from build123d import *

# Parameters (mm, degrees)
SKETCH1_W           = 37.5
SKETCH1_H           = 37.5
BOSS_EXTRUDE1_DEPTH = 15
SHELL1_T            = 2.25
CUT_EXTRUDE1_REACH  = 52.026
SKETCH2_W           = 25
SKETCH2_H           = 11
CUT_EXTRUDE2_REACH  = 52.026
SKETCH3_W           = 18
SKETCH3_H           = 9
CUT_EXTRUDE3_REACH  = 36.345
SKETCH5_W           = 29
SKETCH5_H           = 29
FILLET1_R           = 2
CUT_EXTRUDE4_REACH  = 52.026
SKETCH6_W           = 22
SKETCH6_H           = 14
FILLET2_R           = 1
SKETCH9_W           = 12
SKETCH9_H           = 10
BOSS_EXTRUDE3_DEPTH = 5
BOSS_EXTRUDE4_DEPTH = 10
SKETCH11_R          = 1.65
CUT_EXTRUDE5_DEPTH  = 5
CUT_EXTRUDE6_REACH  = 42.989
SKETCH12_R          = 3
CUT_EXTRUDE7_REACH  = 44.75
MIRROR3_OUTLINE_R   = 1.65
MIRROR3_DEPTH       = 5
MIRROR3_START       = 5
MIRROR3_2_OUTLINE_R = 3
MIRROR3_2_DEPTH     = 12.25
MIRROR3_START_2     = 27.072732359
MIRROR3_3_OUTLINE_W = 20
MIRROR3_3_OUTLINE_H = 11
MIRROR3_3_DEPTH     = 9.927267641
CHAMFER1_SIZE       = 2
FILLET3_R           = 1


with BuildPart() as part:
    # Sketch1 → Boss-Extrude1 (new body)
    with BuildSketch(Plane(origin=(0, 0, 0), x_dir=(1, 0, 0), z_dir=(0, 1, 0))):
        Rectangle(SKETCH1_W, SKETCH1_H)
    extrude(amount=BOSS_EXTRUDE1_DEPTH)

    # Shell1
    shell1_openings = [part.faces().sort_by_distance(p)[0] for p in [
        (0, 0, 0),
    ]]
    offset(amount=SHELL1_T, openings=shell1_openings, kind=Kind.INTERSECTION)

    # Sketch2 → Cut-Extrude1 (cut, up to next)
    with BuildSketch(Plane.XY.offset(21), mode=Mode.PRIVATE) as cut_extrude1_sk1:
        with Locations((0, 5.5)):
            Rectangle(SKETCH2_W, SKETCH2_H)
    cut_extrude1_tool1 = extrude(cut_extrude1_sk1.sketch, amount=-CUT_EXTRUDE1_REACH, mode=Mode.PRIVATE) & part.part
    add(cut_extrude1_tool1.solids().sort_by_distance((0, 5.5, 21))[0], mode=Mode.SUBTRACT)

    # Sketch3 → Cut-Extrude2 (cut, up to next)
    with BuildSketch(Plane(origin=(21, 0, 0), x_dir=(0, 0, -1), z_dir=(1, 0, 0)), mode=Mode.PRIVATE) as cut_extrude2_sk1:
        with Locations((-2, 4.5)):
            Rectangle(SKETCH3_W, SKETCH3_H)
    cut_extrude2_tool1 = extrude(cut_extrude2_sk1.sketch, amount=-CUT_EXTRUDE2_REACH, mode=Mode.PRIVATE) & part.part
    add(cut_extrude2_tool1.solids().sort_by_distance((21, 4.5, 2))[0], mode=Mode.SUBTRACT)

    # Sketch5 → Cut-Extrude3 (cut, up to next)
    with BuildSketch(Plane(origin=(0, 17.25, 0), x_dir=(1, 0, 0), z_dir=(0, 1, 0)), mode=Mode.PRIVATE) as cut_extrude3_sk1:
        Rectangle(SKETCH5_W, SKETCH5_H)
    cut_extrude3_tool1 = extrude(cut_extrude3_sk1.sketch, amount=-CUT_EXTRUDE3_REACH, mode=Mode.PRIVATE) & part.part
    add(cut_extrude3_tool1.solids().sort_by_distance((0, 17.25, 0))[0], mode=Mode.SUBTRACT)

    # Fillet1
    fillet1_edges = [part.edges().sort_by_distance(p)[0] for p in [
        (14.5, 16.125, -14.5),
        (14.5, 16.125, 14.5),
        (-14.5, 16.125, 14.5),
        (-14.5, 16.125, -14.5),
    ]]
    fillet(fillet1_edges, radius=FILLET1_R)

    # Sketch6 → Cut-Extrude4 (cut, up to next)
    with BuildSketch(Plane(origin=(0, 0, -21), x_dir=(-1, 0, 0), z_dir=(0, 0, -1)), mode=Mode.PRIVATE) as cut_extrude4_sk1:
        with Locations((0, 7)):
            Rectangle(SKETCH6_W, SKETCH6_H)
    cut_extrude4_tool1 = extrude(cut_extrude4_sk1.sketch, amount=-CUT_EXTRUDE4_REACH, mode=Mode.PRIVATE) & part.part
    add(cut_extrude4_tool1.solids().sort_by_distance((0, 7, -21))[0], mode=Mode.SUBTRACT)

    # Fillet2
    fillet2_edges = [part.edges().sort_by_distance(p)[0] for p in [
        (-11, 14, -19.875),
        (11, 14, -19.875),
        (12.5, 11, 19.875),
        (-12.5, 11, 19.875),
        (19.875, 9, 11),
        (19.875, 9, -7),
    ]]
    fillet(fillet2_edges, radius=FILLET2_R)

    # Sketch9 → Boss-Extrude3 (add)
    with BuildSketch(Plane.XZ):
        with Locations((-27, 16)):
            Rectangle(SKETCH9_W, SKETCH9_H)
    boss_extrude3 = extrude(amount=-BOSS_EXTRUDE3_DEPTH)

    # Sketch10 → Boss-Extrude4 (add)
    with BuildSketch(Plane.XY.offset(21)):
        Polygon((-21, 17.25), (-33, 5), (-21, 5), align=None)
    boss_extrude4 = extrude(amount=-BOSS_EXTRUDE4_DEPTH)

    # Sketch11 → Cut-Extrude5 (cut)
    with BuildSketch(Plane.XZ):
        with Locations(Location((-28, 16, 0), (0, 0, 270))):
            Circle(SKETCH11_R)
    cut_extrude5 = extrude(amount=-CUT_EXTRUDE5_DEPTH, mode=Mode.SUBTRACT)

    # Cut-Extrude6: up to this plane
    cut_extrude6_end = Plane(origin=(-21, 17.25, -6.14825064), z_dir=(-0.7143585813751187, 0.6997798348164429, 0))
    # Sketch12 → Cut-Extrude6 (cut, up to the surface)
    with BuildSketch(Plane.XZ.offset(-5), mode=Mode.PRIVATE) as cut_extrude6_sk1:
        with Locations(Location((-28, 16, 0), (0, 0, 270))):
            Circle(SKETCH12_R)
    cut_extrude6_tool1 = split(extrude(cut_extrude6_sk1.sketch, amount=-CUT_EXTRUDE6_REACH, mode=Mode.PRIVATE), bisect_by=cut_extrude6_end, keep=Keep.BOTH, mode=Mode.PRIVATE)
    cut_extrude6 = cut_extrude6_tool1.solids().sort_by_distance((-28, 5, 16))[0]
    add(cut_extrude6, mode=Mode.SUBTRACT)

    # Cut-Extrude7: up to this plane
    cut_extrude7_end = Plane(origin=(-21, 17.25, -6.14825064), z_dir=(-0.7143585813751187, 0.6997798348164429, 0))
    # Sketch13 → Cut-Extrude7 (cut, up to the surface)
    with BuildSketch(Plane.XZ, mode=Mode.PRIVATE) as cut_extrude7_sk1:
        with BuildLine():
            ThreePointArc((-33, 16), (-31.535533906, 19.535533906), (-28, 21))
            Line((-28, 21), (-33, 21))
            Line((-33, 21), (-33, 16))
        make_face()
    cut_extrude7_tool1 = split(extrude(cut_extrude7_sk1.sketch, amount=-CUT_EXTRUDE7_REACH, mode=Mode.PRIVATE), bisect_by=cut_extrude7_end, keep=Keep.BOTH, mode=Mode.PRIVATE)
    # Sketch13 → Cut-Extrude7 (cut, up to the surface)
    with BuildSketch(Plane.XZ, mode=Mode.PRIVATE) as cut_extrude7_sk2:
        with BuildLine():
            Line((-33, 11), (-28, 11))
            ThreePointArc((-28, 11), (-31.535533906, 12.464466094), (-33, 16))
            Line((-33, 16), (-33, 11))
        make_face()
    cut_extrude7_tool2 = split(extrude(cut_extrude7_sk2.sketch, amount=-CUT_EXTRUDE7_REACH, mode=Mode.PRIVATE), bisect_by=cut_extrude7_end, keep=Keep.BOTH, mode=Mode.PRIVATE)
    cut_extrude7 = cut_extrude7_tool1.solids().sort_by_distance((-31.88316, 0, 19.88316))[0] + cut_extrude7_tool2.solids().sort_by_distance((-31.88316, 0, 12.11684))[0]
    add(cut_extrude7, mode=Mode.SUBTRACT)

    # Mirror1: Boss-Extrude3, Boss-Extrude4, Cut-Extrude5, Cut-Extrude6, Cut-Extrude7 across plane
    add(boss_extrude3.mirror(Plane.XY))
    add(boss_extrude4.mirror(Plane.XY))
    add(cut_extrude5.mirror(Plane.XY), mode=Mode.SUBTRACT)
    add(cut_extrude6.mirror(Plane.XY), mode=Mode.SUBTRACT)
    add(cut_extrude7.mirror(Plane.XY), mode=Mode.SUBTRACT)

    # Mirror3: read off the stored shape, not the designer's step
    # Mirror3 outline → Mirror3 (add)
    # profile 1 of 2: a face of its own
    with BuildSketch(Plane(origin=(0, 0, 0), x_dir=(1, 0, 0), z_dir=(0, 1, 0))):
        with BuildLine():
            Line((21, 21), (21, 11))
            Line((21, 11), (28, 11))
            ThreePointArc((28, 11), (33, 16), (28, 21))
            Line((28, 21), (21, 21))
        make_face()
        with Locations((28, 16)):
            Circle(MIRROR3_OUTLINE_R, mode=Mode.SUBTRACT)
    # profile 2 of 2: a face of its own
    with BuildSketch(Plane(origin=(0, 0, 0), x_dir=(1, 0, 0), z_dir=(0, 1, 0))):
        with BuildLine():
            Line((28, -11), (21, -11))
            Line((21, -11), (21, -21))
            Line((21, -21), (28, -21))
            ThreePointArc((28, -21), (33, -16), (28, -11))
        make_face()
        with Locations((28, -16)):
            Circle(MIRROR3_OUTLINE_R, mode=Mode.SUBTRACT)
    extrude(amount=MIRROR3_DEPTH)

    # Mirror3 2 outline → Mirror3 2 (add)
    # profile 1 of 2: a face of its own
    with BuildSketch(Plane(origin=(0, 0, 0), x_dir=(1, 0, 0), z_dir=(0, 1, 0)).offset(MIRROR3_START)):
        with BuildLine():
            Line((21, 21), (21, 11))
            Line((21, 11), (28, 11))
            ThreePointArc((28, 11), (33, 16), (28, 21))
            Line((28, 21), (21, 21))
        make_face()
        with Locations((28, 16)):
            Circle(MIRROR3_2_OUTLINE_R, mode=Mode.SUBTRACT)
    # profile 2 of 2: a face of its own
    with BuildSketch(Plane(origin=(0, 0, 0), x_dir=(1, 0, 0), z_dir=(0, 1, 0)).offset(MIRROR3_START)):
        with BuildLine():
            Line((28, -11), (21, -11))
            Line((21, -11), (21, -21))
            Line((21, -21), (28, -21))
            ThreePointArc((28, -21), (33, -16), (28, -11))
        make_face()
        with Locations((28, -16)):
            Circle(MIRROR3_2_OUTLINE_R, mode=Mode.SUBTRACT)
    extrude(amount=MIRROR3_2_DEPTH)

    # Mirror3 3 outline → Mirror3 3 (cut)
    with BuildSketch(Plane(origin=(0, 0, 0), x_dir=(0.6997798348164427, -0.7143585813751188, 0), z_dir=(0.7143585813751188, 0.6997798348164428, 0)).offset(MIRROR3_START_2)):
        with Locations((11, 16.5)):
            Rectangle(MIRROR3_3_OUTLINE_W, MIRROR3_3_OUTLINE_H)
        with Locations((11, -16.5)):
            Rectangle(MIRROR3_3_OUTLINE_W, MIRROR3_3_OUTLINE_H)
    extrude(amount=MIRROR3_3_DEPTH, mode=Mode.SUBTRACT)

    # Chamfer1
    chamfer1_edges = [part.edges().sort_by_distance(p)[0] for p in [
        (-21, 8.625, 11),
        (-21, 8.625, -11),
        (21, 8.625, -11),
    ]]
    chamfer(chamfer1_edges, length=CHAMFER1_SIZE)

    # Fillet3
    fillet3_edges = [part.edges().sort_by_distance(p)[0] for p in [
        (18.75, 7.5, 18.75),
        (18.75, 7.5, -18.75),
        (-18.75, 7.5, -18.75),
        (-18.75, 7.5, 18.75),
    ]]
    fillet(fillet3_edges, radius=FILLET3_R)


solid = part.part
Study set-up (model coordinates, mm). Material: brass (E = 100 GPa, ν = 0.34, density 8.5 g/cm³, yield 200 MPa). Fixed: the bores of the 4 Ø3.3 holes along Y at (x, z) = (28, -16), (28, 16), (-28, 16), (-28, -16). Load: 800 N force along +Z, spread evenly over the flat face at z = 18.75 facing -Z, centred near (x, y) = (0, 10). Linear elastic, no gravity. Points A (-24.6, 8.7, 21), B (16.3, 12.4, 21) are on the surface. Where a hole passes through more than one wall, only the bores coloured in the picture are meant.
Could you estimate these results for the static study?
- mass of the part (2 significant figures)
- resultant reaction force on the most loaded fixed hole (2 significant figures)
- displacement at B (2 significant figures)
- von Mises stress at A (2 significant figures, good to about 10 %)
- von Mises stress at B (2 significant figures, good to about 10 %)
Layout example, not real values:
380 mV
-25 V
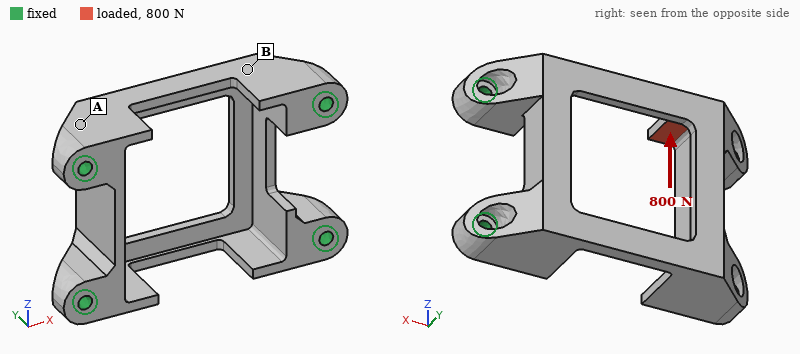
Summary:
87 g
250 N
10 µm
10 MPa
31 MPa
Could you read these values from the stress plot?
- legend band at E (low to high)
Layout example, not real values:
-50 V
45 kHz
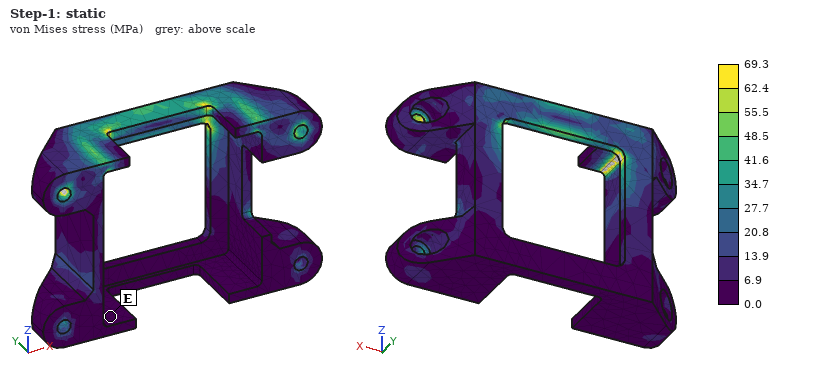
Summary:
0.0 to 6.9 MPa
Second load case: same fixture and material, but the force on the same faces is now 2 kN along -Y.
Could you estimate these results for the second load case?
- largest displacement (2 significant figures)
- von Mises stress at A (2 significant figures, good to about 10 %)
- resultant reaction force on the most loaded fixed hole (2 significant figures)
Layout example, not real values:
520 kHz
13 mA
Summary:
46 µm
15 MPa
1.4 kN
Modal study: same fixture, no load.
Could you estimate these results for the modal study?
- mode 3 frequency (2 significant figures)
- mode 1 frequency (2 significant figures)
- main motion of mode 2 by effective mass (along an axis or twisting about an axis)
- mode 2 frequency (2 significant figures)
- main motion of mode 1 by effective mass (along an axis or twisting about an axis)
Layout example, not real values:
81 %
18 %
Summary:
9300 Hz
7500 Hz
along Z
8400 Hz
along X
